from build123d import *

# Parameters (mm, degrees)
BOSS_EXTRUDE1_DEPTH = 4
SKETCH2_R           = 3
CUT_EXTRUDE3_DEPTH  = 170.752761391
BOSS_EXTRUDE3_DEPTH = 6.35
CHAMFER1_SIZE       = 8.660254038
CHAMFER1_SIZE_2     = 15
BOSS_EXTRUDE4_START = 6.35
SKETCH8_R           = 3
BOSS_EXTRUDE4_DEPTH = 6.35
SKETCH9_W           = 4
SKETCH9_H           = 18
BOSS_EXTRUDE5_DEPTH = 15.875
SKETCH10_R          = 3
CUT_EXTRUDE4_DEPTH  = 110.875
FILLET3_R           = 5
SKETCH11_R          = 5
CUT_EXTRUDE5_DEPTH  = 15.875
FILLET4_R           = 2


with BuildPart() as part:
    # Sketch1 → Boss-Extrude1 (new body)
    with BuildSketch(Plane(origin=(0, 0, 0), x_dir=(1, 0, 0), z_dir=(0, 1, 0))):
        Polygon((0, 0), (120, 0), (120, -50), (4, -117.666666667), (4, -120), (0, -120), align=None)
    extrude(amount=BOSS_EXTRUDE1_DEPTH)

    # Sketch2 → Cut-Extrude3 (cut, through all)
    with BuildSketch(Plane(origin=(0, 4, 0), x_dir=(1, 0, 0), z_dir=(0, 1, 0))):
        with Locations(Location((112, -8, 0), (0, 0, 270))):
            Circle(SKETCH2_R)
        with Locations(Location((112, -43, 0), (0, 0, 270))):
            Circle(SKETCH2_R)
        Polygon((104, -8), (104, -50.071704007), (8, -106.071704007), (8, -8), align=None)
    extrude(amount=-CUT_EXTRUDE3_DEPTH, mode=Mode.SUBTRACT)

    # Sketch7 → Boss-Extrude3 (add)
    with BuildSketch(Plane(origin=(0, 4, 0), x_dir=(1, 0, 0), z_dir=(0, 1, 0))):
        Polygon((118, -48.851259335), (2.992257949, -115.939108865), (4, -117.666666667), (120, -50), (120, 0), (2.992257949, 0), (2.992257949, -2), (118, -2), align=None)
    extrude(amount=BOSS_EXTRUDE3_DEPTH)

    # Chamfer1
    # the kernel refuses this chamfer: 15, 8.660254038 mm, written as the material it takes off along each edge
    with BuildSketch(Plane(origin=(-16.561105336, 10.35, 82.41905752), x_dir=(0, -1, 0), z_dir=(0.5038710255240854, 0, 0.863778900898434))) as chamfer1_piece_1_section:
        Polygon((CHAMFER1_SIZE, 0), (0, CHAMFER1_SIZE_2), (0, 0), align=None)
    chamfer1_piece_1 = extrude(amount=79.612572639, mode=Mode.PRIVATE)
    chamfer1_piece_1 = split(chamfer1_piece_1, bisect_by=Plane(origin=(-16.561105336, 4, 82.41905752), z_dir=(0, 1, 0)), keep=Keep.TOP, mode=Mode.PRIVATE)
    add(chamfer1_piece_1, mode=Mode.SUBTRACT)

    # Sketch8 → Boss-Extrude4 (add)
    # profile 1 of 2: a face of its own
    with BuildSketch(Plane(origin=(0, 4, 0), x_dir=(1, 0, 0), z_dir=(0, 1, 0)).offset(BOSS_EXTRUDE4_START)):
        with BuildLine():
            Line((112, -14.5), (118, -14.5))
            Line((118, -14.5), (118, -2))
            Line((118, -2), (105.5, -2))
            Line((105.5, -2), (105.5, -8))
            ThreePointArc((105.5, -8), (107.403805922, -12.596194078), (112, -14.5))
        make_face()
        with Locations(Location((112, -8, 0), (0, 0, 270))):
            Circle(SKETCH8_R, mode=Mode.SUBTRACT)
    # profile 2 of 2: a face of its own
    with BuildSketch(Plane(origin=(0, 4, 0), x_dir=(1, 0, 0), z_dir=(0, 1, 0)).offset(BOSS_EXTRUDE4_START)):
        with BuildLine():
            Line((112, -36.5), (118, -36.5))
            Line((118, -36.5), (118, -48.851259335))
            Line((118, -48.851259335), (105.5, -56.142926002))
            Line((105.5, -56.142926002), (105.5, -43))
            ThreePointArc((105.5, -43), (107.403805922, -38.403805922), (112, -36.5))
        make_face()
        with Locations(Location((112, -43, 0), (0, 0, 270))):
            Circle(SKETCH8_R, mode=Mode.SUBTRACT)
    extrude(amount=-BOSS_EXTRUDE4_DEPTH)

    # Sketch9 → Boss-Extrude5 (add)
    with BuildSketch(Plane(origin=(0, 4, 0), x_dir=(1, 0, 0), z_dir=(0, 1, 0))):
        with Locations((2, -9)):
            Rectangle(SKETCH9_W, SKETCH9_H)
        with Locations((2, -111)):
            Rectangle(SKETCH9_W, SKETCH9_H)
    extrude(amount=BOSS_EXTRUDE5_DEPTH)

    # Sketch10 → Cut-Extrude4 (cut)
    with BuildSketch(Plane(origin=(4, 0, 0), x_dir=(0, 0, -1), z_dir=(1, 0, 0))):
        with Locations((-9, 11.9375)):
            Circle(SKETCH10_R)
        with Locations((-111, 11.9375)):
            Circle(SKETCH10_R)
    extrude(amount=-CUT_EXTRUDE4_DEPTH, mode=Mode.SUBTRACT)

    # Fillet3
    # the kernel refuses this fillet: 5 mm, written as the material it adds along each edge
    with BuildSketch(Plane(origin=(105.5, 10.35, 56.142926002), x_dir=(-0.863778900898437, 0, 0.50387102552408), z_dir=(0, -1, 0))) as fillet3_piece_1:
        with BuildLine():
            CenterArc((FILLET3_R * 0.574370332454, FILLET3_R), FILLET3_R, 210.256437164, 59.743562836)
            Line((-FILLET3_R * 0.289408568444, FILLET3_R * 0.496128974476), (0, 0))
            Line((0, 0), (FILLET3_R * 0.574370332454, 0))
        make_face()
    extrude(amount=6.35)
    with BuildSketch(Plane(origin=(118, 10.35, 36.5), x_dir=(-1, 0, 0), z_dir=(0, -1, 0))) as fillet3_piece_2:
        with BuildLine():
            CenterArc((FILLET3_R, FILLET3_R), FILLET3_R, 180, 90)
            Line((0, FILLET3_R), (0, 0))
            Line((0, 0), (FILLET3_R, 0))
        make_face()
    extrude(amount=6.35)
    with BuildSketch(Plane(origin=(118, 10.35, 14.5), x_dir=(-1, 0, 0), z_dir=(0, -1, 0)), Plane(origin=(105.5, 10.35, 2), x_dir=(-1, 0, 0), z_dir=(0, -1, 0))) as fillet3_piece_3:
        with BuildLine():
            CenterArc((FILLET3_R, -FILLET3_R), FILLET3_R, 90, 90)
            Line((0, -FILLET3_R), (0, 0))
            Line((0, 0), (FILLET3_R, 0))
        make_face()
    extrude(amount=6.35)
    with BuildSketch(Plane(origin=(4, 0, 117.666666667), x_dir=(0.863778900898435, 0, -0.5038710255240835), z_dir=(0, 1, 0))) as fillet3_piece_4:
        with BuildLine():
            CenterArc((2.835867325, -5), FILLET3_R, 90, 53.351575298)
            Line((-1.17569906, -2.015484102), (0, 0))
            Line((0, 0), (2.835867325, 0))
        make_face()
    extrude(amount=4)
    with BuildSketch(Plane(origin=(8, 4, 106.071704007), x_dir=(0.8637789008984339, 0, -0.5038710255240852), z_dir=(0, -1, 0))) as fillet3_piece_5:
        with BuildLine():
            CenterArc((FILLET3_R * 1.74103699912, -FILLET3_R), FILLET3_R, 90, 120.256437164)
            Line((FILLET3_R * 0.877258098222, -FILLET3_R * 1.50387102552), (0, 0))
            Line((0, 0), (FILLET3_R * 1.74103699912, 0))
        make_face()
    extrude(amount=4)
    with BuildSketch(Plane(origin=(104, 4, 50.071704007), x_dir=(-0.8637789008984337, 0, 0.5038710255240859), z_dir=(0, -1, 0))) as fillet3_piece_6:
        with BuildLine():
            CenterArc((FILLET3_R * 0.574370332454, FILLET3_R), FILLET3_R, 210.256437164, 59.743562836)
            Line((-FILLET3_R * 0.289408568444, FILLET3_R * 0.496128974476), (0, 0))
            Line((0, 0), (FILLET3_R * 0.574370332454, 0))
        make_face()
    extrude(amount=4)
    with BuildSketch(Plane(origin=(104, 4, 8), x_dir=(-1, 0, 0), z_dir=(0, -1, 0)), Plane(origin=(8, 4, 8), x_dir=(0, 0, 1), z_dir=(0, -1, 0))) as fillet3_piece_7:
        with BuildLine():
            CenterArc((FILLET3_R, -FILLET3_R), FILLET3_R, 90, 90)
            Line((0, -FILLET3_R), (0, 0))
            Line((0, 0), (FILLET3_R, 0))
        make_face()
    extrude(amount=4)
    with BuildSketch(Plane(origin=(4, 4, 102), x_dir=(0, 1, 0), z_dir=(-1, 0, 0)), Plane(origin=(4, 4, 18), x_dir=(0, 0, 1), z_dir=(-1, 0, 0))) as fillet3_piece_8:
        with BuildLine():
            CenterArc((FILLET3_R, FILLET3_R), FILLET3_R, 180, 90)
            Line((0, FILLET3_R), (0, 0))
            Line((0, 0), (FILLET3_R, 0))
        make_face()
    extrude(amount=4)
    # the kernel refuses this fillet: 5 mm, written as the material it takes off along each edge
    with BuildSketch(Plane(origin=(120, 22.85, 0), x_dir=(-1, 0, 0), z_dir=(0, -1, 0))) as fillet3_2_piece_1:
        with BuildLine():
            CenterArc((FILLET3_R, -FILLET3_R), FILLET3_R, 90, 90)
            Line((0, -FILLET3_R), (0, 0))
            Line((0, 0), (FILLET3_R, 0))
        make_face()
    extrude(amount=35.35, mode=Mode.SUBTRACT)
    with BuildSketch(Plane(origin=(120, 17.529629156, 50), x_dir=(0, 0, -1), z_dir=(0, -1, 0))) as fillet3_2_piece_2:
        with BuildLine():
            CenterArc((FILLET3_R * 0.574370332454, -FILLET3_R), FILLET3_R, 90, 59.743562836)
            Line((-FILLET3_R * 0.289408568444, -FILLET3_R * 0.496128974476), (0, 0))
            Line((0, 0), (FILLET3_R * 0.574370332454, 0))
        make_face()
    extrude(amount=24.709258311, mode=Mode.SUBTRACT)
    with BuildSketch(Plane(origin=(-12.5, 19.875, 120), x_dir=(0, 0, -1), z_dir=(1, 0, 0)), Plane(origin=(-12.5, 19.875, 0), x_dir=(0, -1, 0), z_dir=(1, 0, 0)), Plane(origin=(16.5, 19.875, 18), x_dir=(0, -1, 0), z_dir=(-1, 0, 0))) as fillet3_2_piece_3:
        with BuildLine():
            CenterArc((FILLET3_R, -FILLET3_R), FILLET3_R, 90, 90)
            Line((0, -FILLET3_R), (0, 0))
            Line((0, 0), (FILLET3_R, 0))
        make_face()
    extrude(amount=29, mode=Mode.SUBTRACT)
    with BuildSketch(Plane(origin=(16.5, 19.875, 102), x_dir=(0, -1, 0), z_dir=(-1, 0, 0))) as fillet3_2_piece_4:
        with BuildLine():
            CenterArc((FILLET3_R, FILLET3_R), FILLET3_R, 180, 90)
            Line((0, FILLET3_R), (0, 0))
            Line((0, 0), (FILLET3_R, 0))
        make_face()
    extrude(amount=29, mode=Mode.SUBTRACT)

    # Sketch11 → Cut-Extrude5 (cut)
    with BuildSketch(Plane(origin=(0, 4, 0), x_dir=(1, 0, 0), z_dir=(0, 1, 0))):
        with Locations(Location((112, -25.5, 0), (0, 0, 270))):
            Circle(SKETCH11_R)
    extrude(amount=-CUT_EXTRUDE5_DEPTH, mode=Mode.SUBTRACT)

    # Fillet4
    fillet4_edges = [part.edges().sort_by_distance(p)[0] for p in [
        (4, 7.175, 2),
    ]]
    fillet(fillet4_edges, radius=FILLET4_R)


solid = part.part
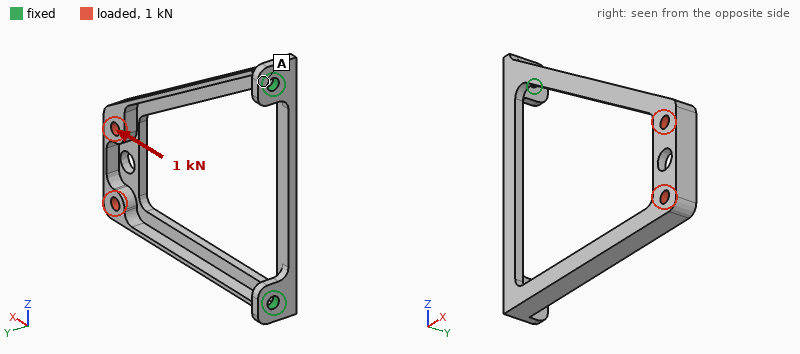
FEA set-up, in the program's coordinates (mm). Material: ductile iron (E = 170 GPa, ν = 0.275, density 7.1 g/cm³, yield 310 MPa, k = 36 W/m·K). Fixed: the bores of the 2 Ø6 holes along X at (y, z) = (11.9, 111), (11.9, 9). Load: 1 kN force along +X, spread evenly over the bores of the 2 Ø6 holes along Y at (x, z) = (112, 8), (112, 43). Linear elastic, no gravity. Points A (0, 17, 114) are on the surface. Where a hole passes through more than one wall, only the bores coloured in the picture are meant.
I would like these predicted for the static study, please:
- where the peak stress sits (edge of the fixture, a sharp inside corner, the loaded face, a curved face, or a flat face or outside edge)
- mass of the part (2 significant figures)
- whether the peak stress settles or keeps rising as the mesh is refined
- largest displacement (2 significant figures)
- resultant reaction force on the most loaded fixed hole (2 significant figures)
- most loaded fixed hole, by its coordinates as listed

edge of the fixture
150 g
keeps rising
0.28 mm
760 N
(11.9, 9)
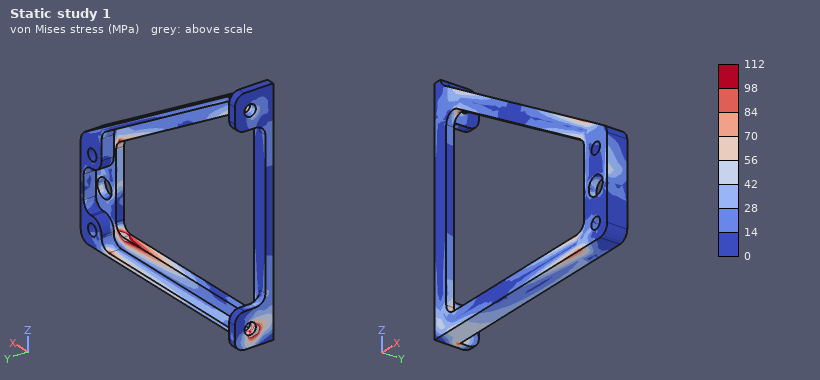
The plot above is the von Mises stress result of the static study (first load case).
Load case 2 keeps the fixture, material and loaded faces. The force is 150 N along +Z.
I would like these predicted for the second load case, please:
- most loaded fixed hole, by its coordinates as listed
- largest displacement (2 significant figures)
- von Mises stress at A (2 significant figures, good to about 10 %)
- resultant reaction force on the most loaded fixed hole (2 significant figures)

(11.9, 111)
0.13 mm
4.6 MPa
160 N
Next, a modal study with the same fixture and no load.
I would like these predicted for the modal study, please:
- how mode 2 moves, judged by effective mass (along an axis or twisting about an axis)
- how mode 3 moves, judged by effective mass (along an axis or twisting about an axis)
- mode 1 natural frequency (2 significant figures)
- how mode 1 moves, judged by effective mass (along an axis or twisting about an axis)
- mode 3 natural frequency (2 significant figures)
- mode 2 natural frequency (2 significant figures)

along Z
along Z
240 Hz
along Y
930 Hz
610 Hz
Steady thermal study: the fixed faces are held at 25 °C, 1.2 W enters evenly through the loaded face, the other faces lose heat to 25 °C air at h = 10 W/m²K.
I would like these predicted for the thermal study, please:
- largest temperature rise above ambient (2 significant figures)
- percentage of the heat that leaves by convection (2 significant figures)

16 K
78 %
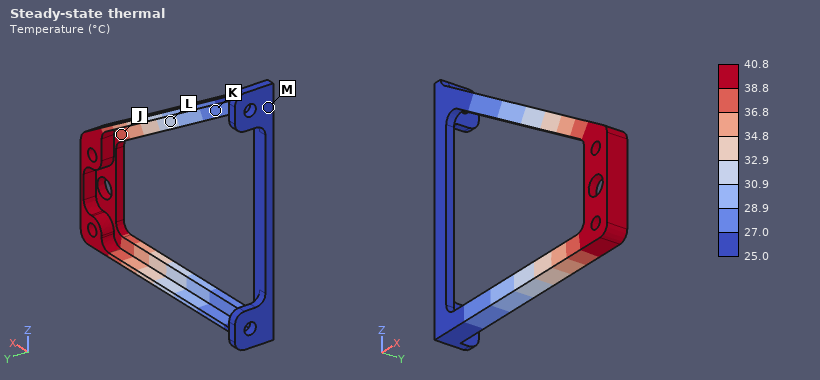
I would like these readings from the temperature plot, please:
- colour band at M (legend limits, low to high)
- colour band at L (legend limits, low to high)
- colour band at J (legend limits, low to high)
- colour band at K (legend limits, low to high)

25.0 to 27.0 °C
30.9 to 32.9 °C
36.8 to 38.8 °C
27.0 to 28.9 °C
